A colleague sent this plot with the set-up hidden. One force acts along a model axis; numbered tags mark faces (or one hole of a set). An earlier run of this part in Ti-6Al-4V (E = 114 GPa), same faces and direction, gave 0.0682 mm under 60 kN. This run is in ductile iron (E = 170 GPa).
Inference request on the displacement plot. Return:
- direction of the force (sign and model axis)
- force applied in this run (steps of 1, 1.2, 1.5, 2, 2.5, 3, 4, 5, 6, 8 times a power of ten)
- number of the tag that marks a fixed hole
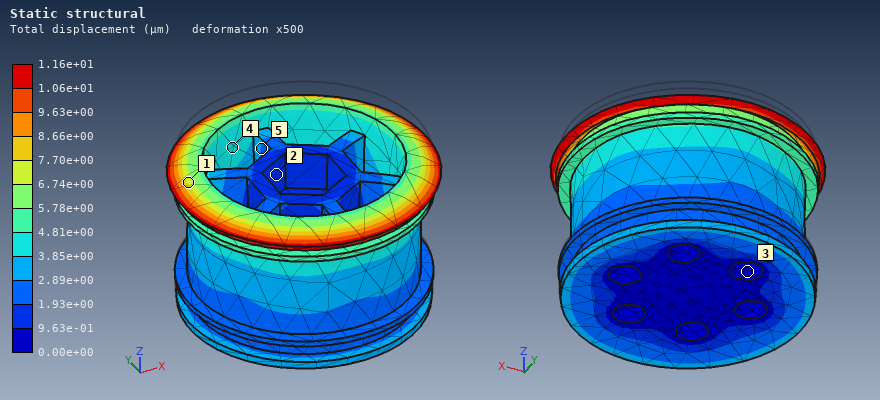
-Z
15 kN
3
